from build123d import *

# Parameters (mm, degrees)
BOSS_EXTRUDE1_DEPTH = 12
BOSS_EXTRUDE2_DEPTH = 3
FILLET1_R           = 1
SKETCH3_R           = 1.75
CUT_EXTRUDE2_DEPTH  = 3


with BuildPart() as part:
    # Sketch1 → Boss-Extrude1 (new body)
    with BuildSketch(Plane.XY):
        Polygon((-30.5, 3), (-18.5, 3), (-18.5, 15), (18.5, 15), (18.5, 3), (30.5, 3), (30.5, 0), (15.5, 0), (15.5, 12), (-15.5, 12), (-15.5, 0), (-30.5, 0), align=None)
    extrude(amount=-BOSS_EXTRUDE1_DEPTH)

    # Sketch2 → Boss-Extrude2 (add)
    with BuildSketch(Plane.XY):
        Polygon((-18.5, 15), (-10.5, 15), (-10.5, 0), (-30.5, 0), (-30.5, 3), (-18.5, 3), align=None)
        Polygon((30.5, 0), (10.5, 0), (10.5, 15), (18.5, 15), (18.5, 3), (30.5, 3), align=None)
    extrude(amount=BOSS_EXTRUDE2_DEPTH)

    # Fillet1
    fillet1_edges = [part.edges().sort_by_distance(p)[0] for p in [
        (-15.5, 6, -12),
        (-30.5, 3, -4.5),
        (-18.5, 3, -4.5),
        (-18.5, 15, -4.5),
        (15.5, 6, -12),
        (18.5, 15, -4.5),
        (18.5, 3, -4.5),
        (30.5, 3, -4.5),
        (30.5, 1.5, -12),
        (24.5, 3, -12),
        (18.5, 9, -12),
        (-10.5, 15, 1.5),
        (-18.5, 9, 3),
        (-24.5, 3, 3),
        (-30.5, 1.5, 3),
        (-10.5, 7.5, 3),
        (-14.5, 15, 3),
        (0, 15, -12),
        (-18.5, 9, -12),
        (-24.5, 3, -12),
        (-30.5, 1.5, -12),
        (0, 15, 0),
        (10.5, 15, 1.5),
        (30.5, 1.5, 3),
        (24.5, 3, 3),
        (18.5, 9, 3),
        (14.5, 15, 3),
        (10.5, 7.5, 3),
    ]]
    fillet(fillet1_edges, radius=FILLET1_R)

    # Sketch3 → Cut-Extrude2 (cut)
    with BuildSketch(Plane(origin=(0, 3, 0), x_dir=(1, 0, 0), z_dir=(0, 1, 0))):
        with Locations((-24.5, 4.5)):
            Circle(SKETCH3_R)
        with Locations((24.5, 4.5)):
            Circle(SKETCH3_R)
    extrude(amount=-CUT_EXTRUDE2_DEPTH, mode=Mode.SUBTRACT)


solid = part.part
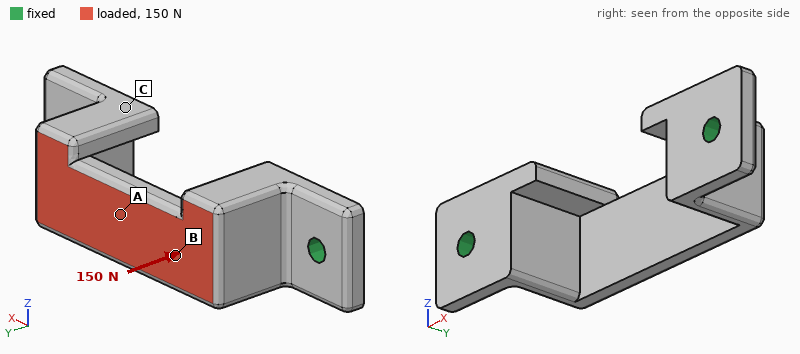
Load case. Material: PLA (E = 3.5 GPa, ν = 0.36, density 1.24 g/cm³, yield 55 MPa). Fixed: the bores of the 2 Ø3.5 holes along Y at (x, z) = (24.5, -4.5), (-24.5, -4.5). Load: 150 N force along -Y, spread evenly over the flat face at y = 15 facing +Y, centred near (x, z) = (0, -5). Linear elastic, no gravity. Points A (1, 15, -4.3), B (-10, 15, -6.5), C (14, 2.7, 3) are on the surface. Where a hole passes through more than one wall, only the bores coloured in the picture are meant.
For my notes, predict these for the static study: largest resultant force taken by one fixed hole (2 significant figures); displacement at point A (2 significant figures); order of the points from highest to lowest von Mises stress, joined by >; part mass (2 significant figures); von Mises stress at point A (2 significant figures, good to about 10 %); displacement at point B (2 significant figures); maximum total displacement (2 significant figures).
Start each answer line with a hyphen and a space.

- 93 N
- 0.17 mm
- A > B > C
- 4.8 g
- 11 MPa
- 0.11 mm
- 0.23 mm
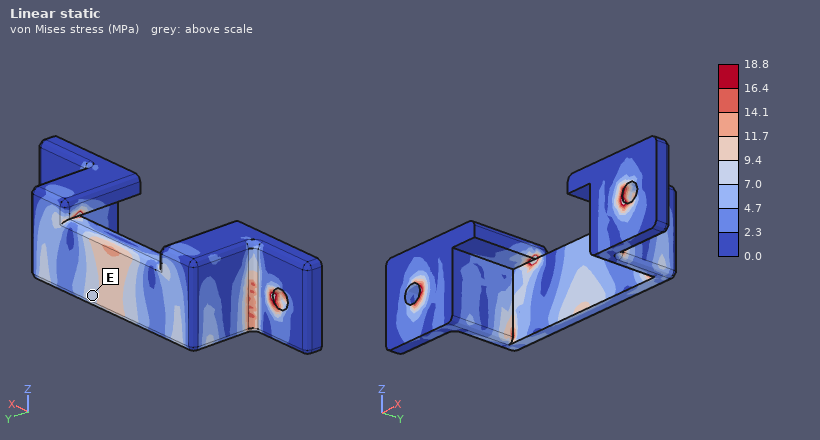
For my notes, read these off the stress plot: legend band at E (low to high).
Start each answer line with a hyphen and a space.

- 7.0 to 9.4 MPa
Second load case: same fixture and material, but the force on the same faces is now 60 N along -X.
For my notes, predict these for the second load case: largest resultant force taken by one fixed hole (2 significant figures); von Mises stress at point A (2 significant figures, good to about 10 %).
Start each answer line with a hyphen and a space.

- 33 N
- 1.5 MPa
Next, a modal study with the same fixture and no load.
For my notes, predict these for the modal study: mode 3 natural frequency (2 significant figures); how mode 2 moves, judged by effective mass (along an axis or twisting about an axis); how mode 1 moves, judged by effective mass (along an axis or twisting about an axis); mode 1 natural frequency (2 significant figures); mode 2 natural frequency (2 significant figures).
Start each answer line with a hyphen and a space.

- 3200 Hz
- along X
- along Z
- 1900 Hz
- 2400 Hz
